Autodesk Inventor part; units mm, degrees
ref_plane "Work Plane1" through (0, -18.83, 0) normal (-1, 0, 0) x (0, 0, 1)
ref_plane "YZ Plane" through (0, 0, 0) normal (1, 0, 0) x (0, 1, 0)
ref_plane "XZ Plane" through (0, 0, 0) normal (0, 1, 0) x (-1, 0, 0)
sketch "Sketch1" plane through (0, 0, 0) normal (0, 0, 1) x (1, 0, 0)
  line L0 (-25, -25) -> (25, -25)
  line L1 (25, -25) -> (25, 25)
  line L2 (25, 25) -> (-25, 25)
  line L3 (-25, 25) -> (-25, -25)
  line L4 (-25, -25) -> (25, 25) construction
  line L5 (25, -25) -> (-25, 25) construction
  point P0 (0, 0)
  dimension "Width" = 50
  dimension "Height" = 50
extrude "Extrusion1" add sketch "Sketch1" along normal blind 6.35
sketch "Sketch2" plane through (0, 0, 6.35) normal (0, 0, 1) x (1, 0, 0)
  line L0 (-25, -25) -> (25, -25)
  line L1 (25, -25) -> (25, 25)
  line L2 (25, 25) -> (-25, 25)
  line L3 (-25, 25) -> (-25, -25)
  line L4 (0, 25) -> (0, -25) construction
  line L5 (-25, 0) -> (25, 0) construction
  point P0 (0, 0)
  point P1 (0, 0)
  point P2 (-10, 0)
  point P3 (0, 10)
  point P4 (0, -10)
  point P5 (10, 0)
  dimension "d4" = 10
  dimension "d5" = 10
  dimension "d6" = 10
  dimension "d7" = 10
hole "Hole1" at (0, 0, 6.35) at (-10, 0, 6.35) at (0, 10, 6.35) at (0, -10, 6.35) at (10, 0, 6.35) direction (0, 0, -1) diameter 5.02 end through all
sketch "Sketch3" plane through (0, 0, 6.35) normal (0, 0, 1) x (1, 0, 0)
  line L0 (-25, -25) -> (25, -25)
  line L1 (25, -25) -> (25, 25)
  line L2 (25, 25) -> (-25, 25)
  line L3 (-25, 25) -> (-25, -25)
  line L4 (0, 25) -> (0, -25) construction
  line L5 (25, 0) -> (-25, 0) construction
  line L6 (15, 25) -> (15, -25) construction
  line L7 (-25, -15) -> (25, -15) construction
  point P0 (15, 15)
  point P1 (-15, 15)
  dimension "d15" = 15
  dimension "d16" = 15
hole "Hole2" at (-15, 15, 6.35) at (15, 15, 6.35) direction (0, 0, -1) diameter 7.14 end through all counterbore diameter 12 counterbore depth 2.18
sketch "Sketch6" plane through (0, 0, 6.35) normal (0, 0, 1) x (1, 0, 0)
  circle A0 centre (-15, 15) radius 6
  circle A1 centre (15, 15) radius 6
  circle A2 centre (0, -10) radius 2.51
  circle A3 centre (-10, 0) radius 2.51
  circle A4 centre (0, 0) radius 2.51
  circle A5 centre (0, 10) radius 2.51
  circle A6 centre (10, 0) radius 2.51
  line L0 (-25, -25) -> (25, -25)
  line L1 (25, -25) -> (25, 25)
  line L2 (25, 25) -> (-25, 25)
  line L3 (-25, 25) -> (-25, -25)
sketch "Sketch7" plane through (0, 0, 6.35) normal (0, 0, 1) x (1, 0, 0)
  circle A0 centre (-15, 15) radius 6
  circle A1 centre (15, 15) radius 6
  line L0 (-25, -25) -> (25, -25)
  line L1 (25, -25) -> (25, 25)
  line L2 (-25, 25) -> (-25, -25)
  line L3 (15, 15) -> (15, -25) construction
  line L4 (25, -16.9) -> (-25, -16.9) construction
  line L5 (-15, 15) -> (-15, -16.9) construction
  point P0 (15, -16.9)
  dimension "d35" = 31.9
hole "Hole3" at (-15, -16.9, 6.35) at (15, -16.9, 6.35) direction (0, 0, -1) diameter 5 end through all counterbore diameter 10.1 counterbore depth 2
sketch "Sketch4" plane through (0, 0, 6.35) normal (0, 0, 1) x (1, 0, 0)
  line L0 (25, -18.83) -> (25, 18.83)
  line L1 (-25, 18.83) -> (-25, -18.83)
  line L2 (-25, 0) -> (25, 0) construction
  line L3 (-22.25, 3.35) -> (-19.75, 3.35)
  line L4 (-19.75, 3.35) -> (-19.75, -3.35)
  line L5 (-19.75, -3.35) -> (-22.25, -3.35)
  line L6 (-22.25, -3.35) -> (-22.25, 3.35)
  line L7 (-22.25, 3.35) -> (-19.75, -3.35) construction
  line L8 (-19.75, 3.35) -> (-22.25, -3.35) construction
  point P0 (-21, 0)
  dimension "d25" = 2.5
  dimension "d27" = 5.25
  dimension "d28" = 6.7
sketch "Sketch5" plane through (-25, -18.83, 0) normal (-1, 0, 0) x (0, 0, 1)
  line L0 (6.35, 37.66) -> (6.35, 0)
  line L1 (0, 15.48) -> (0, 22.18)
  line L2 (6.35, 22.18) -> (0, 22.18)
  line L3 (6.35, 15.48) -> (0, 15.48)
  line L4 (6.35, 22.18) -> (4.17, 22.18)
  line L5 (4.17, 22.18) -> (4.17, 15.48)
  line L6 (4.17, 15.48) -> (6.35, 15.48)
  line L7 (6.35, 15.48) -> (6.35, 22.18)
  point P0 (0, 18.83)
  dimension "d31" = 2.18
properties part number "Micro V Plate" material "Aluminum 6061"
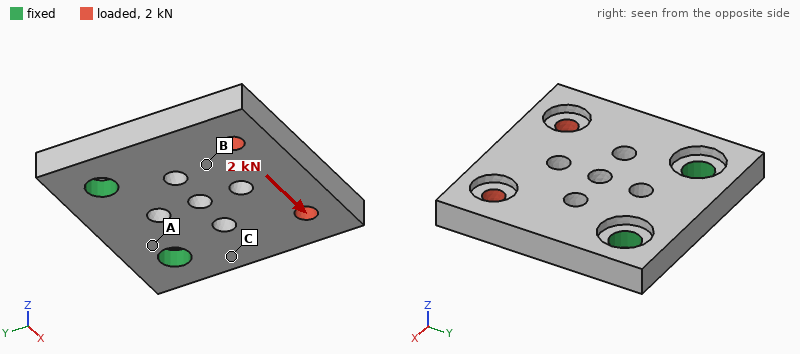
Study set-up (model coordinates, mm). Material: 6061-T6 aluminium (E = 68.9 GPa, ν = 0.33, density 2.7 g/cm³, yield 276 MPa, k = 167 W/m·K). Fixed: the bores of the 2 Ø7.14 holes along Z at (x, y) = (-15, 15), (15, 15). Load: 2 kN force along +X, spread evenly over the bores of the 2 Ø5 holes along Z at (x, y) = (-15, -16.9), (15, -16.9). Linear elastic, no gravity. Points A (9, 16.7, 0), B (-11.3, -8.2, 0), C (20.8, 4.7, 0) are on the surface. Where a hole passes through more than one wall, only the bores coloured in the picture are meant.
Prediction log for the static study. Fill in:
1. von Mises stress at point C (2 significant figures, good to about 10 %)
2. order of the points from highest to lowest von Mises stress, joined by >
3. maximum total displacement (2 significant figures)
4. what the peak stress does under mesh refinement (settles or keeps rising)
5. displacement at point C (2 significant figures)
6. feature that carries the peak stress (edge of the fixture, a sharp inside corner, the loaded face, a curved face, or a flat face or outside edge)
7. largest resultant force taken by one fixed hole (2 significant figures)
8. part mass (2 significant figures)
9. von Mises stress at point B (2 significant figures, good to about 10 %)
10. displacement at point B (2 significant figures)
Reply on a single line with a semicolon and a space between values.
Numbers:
17 MPa; B > C > A; 33 µm; keeps rising; 8.1 µm; edge of the fixture; 2.0 kN; 38 g; 25 MPa; 17 µm
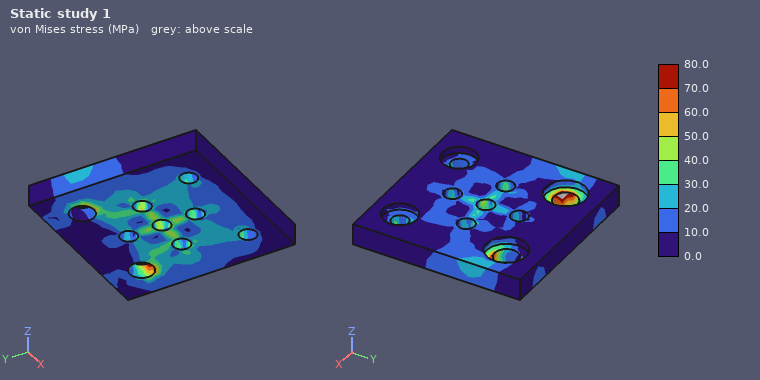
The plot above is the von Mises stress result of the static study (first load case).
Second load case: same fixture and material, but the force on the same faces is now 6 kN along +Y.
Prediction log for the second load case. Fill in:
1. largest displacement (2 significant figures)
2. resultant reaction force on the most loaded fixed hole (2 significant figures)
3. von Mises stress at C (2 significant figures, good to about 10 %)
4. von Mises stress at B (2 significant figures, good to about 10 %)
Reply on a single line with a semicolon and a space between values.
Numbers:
56 µm; 3.0 kN; 42 MPa; 37 MPa
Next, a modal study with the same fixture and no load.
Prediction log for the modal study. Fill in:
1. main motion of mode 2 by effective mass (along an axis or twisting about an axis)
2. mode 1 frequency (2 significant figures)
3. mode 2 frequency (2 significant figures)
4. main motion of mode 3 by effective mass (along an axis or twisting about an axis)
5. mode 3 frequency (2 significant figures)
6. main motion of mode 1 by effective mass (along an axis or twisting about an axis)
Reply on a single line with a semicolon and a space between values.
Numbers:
twisting about Y; 2800 Hz; 5800 Hz; along X; 12 kHz; along Z
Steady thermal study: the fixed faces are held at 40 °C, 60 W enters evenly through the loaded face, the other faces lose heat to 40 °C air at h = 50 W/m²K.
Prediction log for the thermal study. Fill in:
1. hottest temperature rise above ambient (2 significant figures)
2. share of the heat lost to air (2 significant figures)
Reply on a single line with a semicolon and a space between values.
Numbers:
47 K; 11 %
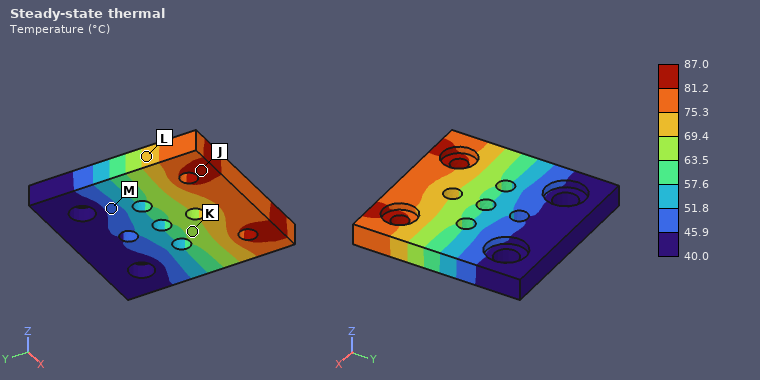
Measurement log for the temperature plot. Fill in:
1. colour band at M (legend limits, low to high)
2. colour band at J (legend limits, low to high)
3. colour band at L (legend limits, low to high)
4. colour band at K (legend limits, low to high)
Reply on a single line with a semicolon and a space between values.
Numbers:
45.9 to 51.8 °C; 81.2 to 87.0 °C; 69.4 to 75.3 °C; 63.5 to 69.4 °C
